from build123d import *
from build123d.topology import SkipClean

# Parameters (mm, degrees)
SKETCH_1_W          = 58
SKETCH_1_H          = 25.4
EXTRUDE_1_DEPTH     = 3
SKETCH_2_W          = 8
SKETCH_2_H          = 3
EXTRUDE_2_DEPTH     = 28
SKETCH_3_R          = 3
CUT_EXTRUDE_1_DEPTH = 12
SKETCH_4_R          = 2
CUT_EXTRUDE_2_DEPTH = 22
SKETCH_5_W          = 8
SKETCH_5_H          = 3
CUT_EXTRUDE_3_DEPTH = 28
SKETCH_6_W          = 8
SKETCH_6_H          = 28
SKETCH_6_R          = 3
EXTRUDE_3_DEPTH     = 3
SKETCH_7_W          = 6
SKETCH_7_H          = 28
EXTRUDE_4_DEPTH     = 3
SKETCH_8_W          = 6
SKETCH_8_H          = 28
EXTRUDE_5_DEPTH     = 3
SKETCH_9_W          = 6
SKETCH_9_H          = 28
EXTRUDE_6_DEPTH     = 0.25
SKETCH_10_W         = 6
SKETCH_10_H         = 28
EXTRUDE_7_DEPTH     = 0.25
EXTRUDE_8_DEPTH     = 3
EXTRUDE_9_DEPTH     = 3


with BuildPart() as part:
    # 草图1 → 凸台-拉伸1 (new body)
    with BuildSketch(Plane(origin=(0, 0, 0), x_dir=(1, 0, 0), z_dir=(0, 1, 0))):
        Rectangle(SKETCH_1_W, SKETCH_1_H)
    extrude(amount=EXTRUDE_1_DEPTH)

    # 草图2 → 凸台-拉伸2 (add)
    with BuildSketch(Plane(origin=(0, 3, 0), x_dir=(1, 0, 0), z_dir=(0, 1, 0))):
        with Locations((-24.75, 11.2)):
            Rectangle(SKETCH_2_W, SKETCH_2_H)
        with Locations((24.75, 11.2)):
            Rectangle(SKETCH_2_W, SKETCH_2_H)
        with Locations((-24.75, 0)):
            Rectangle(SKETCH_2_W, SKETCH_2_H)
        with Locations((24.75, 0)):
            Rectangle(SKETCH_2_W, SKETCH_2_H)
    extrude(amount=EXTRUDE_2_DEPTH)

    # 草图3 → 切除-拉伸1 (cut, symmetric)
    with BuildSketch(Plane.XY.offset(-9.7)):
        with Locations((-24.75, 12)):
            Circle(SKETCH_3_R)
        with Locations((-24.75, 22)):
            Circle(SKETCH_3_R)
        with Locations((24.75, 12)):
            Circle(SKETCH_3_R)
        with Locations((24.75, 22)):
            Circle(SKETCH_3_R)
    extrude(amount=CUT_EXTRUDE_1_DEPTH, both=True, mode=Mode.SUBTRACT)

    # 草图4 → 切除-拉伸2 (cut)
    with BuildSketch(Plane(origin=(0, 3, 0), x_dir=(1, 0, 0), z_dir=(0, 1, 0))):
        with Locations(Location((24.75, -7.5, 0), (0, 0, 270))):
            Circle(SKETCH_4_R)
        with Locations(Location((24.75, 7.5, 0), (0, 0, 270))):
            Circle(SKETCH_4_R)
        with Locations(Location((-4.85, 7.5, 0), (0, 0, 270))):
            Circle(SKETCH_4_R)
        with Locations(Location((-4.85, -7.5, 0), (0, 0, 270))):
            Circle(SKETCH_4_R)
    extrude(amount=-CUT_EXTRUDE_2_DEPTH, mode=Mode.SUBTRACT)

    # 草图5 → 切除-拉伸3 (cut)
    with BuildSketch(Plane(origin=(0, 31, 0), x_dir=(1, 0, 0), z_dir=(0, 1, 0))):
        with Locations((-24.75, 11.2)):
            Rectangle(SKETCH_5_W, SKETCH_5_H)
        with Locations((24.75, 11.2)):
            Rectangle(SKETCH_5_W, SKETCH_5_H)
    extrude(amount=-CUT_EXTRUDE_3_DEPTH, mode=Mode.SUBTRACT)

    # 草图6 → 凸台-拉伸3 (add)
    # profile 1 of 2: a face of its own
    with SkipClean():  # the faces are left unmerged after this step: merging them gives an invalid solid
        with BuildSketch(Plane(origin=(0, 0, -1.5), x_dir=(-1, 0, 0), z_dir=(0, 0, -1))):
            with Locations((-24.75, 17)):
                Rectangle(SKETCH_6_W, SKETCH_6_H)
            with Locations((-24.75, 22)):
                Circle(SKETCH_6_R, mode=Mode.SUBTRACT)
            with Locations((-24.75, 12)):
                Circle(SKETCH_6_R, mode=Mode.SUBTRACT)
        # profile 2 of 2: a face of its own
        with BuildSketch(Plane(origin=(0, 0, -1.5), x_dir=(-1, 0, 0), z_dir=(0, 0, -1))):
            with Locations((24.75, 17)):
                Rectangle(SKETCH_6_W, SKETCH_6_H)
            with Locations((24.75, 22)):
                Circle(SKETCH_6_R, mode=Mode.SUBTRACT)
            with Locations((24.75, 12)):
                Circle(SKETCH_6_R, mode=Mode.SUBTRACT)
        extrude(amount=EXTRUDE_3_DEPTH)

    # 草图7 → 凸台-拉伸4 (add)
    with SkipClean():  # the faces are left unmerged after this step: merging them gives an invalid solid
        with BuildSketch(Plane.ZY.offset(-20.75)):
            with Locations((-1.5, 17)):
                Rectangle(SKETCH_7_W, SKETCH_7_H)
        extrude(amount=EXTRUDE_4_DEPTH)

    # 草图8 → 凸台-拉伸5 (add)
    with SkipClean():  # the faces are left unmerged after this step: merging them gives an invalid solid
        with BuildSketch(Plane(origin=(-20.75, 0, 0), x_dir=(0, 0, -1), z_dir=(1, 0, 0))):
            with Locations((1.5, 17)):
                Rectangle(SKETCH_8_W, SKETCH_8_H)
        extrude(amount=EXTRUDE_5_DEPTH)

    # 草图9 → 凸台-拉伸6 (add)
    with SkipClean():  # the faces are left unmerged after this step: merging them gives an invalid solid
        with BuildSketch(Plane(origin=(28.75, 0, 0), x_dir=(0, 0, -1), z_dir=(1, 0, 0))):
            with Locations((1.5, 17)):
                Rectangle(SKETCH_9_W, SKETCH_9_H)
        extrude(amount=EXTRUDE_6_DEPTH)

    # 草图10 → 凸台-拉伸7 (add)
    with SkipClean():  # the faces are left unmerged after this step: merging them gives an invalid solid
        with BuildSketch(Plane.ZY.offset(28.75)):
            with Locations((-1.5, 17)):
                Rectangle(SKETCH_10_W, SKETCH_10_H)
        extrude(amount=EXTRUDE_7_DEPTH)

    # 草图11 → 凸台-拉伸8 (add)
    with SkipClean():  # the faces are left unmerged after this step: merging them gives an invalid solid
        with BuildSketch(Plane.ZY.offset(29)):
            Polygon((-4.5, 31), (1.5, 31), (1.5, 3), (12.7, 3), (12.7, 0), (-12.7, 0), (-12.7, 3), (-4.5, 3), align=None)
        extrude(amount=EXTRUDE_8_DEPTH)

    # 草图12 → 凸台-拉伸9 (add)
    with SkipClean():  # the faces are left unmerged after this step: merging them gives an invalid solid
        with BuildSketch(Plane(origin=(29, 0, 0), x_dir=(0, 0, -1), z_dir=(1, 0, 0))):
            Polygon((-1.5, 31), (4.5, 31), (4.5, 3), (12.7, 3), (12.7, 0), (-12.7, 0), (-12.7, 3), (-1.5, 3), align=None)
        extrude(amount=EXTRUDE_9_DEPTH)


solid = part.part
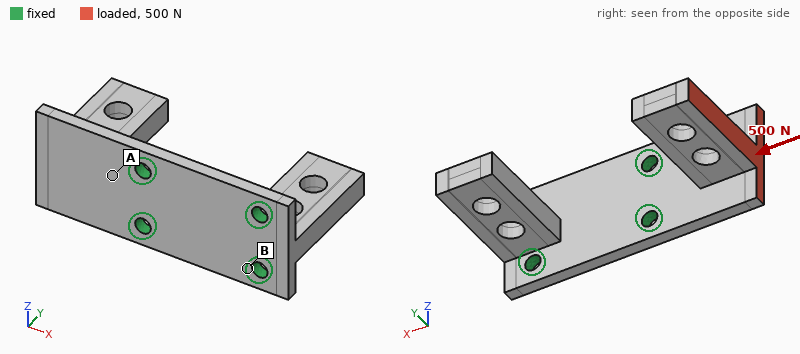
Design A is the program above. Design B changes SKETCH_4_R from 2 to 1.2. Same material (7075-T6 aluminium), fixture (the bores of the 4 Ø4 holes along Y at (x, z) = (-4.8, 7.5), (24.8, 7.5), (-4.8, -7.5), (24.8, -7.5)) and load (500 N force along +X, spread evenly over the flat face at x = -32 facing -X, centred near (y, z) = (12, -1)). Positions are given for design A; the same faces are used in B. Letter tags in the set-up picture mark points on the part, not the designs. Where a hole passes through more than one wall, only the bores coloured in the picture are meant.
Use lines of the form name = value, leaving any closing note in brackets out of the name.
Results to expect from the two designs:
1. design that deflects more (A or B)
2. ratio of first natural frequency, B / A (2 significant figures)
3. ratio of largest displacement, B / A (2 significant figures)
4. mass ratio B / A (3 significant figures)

design that deflects more = B
ratio of first natural frequency, B / A = 0.94
ratio of largest displacement, B / A = 1.1
mass ratio B / A = 1.01
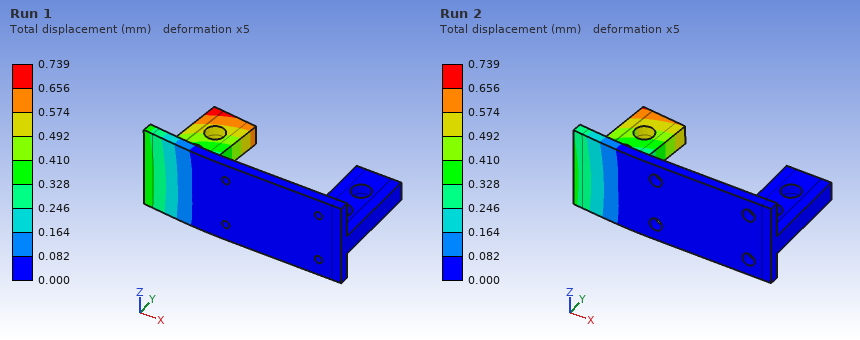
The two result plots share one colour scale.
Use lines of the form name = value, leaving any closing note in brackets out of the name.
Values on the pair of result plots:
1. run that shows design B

run that shows design B = Run 1
